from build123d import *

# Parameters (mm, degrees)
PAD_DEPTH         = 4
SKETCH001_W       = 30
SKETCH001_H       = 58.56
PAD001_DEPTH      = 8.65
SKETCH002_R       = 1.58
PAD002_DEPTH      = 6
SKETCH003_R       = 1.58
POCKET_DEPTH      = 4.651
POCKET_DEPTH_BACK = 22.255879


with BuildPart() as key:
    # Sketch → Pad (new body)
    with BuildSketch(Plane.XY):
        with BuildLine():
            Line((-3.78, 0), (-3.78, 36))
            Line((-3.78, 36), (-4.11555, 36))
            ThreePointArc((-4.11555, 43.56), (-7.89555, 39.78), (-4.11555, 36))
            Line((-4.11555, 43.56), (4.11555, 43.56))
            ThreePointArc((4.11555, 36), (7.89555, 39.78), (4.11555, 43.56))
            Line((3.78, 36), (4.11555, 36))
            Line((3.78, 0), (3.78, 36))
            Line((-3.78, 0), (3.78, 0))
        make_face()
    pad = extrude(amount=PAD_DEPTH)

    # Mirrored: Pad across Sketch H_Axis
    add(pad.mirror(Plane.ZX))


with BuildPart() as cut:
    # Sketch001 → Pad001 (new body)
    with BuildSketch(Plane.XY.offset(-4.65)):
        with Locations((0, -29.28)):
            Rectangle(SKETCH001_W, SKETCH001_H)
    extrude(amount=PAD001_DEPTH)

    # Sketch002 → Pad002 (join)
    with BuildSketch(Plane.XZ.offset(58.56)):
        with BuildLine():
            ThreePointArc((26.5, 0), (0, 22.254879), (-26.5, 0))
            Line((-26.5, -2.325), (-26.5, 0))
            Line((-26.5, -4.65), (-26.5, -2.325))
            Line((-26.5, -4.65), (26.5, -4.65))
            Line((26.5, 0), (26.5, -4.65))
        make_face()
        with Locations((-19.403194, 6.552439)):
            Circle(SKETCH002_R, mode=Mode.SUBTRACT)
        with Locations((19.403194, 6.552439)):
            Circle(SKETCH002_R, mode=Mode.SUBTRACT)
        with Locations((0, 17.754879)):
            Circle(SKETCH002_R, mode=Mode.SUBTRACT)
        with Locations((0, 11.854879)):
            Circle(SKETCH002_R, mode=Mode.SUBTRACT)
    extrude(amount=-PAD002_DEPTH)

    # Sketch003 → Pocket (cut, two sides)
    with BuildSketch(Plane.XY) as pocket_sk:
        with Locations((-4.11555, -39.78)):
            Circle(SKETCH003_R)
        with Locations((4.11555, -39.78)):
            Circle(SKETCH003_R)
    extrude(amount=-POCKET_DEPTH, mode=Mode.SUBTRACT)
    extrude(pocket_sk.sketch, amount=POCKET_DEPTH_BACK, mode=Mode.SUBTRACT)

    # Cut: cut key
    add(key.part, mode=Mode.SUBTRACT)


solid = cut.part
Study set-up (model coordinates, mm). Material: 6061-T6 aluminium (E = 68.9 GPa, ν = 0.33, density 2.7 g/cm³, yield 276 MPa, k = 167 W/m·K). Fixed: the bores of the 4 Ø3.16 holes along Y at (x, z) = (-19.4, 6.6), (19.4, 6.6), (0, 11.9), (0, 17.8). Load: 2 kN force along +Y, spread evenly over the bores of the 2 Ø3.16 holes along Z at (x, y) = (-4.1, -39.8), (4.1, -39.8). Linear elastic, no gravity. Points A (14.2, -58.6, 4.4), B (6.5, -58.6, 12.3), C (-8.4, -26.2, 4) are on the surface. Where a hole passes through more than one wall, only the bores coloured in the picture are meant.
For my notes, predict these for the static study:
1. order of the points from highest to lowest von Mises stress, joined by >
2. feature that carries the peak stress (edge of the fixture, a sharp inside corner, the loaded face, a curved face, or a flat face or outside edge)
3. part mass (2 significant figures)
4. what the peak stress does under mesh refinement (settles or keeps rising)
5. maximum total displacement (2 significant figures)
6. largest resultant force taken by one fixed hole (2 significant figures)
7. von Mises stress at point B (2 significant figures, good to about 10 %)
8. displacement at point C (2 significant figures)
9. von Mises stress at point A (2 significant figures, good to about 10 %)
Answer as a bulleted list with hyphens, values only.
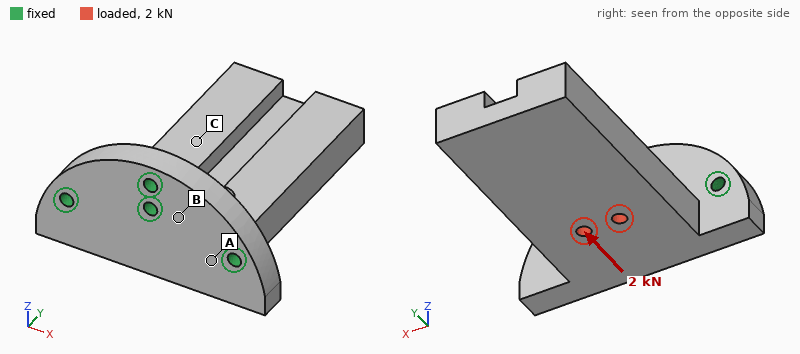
- A > B > C
- edge of the fixture
- 50 g
- keeps rising
- 0.15 mm
- 890 N
- 22 MPa
- 0.076 mm
- 37 MPa
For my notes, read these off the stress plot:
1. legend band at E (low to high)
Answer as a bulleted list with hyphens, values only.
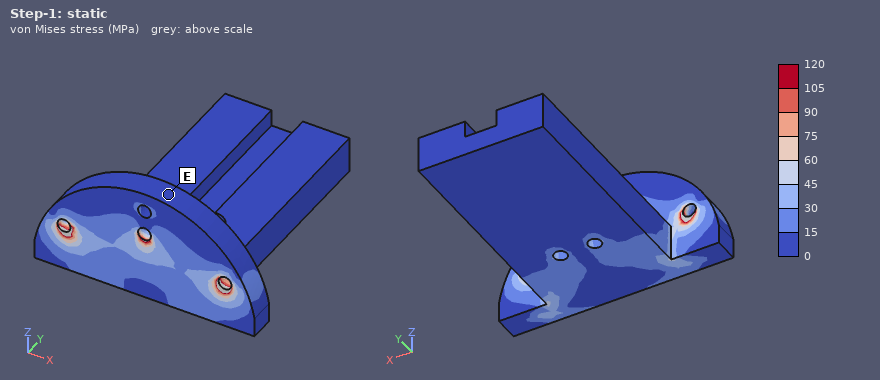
- 0 to 15 MPa
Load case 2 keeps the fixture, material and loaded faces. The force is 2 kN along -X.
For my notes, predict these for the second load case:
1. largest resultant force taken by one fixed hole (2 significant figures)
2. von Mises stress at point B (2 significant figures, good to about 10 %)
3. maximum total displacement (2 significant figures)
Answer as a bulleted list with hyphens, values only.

- 1.3 kN
- 8.5 MPa
- 46 µm
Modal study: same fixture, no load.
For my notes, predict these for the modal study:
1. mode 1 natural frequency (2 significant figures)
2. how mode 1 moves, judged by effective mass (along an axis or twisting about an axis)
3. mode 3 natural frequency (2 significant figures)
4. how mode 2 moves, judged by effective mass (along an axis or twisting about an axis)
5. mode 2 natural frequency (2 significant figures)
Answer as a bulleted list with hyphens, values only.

- 1600 Hz
- along Z
- 6500 Hz
- along X
- 4300 Hz
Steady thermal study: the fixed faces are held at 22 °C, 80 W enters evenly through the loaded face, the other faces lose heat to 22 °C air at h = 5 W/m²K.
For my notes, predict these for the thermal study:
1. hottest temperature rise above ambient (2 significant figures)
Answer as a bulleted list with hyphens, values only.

- 60 K
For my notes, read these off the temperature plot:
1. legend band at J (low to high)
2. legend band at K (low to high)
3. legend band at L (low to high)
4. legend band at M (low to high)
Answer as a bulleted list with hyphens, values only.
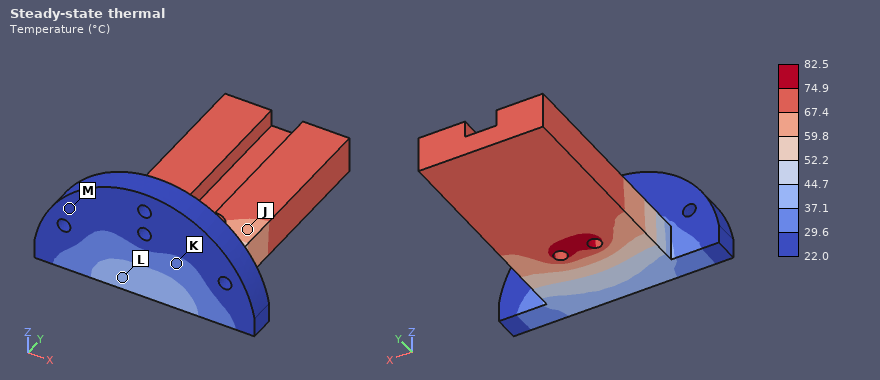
- 59.8 to 67.4 °C
- 29.6 to 37.1 °C
- 37.1 to 44.7 °C
- 22.0 to 29.6 °C
